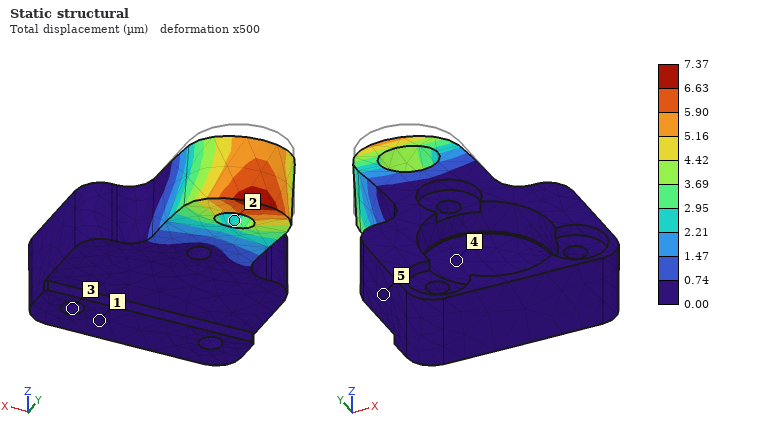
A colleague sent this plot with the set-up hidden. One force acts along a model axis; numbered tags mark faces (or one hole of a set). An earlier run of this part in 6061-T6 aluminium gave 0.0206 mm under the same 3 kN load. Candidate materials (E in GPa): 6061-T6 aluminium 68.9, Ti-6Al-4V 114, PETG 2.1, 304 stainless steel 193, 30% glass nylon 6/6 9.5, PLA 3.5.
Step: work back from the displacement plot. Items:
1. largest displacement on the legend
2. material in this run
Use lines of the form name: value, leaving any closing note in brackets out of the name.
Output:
largest displacement on the legend: 7.37 µm
material in this run: 304 stainless steel
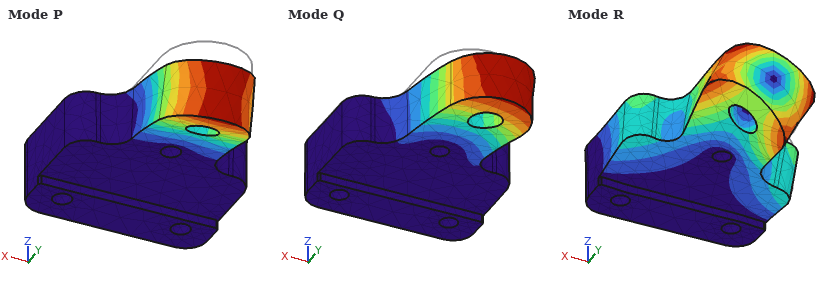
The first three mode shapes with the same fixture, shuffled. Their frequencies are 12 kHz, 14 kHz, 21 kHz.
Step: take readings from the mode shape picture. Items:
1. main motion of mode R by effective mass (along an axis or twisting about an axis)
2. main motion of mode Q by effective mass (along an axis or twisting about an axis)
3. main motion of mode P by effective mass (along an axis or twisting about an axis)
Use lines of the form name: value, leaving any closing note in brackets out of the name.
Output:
main motion of mode R by effective mass: twisting about Y
main motion of mode Q by effective mass: along X
main motion of mode P by effective mass: along Z
